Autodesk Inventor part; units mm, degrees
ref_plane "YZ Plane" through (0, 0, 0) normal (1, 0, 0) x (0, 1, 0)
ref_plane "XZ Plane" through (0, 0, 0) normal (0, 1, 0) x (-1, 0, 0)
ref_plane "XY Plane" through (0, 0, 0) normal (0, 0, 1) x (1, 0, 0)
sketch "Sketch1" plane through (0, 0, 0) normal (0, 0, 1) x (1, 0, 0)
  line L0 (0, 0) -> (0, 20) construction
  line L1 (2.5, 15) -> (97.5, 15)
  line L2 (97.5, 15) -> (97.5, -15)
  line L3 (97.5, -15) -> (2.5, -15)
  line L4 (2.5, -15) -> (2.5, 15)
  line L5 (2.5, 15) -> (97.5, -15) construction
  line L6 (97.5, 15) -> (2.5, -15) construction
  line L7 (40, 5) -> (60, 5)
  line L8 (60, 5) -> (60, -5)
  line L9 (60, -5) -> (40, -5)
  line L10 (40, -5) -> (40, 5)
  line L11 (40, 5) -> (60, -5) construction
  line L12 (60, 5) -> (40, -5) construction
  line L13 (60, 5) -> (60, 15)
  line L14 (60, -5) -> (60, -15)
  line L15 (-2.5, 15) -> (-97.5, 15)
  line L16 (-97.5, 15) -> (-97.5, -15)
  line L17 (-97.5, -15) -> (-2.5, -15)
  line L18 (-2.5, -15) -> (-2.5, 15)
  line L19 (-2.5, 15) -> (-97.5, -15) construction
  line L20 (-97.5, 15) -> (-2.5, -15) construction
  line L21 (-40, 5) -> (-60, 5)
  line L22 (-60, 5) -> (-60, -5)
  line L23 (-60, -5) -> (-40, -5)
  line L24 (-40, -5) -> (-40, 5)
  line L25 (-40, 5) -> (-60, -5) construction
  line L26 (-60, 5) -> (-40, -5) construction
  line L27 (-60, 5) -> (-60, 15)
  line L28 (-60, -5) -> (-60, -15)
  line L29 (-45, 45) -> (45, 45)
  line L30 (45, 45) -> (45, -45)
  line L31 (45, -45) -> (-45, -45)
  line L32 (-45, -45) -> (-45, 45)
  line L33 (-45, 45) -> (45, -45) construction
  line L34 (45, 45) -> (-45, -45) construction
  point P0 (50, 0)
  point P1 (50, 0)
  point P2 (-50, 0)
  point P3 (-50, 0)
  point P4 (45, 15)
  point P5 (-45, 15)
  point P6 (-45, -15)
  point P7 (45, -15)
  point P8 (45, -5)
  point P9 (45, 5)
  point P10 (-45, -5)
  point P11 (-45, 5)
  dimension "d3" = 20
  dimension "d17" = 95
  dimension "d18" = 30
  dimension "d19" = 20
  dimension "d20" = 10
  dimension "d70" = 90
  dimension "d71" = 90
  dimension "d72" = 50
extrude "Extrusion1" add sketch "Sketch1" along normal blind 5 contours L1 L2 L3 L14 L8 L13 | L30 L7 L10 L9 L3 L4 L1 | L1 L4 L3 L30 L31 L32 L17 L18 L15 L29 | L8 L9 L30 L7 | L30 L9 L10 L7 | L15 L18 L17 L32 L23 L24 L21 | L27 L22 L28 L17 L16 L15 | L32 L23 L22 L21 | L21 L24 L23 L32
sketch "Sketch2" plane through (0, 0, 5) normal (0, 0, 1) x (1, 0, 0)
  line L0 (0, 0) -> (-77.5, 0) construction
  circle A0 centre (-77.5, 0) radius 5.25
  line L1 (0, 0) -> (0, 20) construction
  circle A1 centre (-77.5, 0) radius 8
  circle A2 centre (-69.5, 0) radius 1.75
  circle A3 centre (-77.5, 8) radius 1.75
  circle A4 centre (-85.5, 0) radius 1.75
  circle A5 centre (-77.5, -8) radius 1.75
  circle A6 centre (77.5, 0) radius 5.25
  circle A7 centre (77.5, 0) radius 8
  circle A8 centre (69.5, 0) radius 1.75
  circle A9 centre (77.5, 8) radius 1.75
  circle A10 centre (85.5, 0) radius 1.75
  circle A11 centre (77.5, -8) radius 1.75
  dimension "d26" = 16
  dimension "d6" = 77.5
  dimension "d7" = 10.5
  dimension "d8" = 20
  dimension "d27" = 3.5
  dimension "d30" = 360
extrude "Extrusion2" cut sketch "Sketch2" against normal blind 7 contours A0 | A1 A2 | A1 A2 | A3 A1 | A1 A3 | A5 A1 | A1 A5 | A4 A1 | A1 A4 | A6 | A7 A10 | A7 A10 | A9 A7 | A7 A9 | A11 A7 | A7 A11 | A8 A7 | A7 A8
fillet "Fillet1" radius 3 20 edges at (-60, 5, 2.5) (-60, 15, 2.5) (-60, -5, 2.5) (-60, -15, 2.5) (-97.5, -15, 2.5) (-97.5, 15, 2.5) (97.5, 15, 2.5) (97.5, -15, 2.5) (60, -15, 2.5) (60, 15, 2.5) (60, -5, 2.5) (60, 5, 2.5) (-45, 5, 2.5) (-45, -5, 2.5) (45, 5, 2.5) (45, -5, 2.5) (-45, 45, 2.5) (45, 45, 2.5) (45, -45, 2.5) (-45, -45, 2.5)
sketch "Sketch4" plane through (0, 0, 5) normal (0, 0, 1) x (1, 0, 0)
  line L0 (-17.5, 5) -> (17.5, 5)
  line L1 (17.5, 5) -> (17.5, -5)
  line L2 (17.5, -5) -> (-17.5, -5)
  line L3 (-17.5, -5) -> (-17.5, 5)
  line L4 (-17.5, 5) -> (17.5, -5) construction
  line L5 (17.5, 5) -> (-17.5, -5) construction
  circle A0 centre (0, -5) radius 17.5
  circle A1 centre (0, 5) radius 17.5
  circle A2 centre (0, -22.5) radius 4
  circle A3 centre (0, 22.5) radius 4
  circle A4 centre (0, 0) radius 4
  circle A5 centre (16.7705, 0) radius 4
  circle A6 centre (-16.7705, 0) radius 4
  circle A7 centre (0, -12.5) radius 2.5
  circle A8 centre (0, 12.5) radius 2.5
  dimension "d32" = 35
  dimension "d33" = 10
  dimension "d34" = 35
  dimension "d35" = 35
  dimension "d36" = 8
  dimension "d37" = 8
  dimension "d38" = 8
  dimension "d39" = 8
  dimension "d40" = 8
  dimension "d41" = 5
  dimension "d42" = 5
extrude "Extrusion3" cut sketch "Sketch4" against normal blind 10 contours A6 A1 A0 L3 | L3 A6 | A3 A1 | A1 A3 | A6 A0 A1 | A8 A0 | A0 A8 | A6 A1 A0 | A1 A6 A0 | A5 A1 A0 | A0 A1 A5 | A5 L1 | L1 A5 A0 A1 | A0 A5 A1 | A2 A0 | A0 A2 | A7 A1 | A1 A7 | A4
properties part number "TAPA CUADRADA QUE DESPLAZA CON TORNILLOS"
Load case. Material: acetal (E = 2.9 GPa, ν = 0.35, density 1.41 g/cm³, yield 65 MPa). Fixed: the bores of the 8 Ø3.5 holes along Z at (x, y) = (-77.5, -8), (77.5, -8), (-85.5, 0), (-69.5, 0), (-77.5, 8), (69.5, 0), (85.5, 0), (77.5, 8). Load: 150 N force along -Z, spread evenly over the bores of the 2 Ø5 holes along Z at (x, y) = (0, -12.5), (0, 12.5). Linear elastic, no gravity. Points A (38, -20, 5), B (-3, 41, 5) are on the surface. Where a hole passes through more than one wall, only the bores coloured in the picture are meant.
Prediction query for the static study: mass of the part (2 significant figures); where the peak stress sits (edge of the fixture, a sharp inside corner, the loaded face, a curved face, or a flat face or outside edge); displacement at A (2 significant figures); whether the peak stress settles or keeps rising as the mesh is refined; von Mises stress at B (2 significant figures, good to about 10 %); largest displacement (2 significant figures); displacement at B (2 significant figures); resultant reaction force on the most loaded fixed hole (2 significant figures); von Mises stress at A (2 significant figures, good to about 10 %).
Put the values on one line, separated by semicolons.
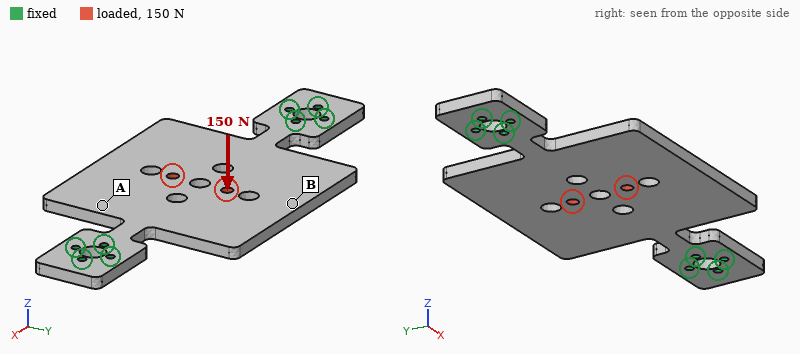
71 g; edge of the fixture; 1.2 mm; keeps rising; 8.6 MPa; 2.1 mm; 2.1 mm; 140 N; 4.2 MPa
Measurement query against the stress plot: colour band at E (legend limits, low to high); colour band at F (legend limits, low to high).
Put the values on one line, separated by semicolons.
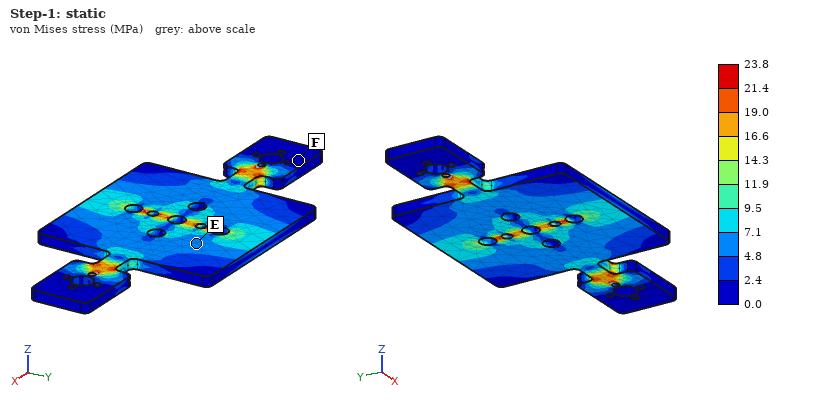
4.8 to 7.1 MPa; 0.0 to 2.4 MPa
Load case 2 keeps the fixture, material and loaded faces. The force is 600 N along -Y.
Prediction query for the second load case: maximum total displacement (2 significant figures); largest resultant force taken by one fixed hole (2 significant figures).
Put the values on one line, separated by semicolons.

0.36 mm; 300 N
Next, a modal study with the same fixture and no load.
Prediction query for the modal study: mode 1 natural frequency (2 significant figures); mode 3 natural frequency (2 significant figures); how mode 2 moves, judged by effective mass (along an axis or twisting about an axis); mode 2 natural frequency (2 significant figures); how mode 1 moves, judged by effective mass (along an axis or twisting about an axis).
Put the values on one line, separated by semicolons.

130 Hz; 540 Hz; along Z; 210 Hz; twisting about X
